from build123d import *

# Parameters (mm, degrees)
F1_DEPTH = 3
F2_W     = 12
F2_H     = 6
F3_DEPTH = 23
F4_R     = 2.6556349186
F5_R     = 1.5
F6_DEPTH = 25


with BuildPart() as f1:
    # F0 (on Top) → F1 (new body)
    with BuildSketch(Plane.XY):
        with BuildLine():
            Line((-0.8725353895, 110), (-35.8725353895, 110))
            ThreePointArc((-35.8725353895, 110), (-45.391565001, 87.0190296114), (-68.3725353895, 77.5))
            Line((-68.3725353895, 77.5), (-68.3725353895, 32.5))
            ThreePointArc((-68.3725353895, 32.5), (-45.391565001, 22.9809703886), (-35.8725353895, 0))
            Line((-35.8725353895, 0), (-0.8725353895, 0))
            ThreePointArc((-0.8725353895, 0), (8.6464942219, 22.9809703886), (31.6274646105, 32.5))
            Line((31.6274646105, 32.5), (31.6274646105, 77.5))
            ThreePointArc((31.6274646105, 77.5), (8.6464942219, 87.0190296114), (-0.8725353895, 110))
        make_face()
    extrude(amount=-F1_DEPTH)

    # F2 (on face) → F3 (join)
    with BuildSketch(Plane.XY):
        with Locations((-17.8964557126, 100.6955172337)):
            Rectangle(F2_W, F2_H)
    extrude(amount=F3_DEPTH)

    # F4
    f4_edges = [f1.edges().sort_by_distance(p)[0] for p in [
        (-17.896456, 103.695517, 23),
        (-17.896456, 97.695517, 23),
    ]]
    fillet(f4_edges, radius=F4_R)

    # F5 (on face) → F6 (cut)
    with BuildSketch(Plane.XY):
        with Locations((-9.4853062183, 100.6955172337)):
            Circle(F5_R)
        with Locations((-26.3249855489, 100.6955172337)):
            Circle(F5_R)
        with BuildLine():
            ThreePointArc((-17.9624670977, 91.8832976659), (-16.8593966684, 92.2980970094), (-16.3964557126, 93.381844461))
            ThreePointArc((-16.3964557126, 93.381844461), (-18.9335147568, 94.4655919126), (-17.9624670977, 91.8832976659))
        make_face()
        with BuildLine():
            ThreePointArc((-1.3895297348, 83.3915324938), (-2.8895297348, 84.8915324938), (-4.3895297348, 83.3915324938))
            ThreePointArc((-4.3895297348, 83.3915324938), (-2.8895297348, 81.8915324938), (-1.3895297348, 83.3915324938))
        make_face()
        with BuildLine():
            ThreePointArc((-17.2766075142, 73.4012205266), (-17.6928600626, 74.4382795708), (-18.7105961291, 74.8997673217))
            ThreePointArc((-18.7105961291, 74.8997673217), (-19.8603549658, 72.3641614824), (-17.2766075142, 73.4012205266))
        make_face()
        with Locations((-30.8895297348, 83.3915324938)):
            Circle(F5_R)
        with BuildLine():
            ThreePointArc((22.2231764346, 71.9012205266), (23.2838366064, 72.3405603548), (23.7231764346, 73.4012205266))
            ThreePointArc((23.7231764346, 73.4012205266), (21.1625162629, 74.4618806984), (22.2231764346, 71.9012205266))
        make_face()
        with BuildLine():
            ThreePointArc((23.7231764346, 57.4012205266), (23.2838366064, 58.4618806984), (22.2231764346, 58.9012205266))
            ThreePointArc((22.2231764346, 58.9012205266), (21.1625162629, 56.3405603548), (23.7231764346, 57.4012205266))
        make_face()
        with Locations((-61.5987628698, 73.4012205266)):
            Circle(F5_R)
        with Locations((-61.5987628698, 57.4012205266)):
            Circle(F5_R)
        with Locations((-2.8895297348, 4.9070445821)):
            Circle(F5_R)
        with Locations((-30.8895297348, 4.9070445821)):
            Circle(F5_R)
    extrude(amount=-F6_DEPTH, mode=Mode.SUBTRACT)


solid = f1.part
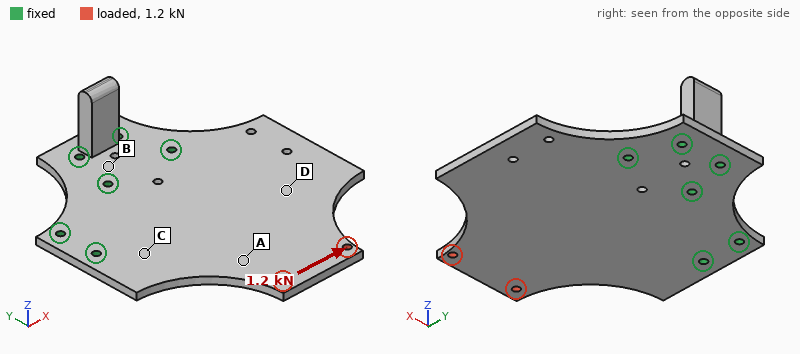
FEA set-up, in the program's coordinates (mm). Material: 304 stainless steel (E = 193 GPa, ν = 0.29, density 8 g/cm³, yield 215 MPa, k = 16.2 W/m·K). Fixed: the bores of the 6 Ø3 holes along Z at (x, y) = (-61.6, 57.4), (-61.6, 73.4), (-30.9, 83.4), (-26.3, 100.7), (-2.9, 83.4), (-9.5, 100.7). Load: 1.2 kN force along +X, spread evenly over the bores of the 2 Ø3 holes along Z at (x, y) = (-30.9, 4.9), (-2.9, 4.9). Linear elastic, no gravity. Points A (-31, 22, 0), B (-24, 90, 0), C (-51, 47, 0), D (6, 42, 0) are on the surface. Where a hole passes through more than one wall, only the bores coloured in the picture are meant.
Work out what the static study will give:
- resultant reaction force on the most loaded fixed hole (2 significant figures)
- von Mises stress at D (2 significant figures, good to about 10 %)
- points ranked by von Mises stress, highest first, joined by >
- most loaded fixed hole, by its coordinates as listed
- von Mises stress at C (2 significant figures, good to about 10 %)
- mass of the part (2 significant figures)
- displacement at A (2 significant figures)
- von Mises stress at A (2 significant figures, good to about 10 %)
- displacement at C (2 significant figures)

1.2 kN
11 MPa
C > A > D > B
(-61.6, 57.4)
21 MPa
200 g
7.1 µm
14 MPa
2.5 µm
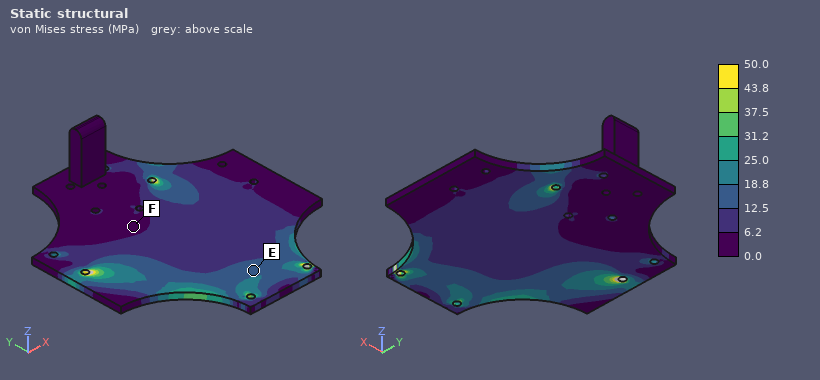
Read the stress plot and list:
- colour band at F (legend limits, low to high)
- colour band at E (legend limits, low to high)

0.0 to 6.2 MPa
12.5 to 18.8 MPa
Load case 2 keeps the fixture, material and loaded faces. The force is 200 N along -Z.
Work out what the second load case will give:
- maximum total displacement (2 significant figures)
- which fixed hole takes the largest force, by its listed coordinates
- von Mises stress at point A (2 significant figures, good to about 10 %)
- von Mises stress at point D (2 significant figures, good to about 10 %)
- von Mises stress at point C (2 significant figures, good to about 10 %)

0.78 mm
(-61.6, 57.4)
59 MPa
42 MPa
77 MPa
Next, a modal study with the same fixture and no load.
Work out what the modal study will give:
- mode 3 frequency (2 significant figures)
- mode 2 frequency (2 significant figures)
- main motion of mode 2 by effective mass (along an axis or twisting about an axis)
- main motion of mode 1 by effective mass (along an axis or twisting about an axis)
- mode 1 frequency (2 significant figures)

2600 Hz
1200 Hz
twisting about Y
along Z
530 Hz
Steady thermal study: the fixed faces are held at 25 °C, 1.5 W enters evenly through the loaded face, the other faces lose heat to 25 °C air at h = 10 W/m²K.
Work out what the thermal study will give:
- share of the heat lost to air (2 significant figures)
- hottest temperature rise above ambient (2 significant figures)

60 %
31 K
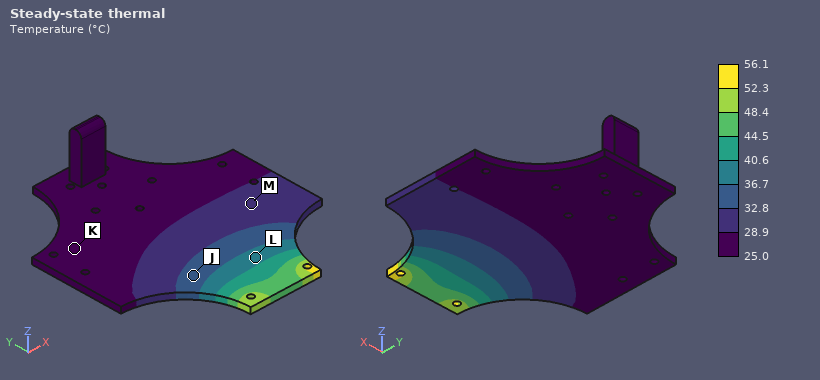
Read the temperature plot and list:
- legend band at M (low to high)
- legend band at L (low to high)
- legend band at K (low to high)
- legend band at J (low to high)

28.9 to 32.8 °C
36.7 to 40.6 °C
25.0 to 28.9 °C
32.8 to 36.7 °C
